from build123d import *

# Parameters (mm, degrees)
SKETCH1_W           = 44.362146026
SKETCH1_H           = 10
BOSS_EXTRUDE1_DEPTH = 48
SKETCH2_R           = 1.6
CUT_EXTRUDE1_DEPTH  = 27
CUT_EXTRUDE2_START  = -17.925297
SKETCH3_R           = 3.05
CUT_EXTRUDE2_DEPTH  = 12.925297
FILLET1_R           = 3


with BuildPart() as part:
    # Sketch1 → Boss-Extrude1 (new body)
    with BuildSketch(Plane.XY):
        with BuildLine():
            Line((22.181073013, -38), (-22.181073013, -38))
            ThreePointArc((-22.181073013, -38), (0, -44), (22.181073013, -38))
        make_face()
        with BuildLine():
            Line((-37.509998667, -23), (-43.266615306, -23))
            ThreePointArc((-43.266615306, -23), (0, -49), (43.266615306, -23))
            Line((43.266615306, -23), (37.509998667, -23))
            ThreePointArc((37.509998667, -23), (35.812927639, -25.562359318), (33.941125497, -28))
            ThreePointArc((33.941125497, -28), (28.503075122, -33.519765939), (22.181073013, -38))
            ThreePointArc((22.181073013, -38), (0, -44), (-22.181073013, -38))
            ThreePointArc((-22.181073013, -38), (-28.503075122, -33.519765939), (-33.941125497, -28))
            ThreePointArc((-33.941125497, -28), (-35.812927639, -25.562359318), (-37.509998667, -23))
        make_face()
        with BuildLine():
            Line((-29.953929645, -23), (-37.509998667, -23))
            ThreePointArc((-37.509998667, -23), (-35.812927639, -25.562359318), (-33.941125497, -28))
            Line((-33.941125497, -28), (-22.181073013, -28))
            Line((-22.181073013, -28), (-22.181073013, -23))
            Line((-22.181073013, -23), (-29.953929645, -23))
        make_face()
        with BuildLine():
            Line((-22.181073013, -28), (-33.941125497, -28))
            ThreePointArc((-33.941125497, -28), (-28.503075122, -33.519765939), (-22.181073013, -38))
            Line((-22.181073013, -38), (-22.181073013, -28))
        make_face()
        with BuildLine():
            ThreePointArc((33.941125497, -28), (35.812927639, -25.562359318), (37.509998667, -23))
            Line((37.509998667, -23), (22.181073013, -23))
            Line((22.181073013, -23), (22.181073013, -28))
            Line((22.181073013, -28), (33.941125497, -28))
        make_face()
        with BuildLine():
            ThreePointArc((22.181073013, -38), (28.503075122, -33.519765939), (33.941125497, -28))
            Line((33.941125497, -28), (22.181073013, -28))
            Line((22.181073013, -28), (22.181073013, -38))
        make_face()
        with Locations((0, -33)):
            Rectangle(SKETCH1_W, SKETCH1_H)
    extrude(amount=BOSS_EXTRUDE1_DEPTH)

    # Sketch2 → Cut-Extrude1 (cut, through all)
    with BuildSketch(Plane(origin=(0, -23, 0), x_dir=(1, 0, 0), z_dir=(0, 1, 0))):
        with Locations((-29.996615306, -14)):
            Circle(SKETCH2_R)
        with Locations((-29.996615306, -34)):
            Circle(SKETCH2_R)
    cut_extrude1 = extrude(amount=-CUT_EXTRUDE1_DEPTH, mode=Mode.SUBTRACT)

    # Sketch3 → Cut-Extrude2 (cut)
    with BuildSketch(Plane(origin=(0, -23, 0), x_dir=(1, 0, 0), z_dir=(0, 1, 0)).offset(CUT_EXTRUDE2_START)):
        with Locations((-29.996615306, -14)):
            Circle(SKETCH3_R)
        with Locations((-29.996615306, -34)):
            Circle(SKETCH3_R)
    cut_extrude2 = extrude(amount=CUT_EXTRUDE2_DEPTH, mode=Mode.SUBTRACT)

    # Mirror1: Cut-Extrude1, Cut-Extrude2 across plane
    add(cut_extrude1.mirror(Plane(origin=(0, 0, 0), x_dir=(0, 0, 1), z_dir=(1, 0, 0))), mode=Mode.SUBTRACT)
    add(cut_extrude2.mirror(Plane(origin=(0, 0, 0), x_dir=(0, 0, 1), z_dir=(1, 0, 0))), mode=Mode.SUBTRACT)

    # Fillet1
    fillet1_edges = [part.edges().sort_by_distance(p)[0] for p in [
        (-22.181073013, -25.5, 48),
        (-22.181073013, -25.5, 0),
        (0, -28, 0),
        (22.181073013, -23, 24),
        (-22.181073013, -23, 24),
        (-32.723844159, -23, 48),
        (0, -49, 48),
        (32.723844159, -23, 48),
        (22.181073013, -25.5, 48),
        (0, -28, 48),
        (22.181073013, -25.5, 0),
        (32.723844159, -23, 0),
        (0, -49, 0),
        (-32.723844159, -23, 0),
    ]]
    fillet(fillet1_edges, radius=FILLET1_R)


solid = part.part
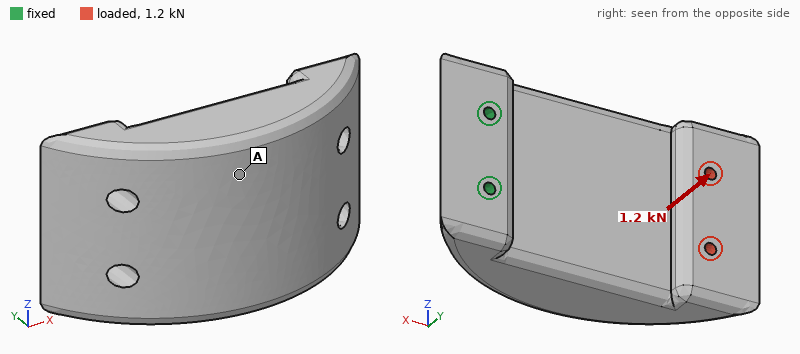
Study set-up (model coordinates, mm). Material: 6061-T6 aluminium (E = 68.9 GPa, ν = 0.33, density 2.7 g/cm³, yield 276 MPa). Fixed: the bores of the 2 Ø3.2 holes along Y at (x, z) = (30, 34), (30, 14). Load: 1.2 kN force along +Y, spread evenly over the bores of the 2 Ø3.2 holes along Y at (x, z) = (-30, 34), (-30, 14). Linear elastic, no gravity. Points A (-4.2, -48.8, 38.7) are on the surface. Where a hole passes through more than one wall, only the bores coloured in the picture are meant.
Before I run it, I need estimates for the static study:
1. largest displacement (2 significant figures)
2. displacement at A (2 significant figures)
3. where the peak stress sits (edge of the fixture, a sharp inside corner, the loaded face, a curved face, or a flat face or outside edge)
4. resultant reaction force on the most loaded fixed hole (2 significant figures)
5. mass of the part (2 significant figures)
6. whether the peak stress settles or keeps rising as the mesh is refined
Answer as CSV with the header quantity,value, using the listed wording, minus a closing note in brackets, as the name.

quantity,value
largest displacement,0.64 mm
displacement at A,0.34 mm
where the peak stress sits,edge of the fixture
resultant reaction force on the most loaded fixed hole,690 N
mass of the part,170 g
whether the peak stress settles or keeps rising as the mesh is refined,keeps rising
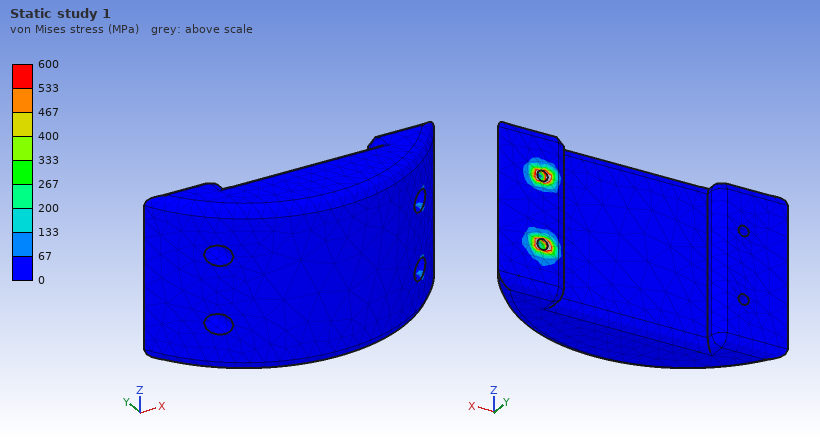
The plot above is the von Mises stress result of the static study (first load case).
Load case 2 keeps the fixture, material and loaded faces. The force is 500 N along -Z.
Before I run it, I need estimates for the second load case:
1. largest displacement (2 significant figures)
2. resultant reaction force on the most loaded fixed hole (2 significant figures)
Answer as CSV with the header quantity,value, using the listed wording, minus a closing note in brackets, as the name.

quantity,value
largest displacement,40 µm
resultant reaction force on the most loaded fixed hole,1.4 kN
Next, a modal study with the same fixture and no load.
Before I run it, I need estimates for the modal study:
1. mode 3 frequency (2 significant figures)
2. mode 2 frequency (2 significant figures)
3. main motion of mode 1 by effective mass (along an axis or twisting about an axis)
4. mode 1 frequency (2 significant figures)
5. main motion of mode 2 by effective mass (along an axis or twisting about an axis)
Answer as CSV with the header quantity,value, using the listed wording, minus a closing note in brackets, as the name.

quantity,value
mode 3 frequency,5200 Hz
mode 2 frequency,2600 Hz
main motion of mode 1 by effective mass,along Y
mode 1 frequency,930 Hz
main motion of mode 2 by effective mass,along Z
